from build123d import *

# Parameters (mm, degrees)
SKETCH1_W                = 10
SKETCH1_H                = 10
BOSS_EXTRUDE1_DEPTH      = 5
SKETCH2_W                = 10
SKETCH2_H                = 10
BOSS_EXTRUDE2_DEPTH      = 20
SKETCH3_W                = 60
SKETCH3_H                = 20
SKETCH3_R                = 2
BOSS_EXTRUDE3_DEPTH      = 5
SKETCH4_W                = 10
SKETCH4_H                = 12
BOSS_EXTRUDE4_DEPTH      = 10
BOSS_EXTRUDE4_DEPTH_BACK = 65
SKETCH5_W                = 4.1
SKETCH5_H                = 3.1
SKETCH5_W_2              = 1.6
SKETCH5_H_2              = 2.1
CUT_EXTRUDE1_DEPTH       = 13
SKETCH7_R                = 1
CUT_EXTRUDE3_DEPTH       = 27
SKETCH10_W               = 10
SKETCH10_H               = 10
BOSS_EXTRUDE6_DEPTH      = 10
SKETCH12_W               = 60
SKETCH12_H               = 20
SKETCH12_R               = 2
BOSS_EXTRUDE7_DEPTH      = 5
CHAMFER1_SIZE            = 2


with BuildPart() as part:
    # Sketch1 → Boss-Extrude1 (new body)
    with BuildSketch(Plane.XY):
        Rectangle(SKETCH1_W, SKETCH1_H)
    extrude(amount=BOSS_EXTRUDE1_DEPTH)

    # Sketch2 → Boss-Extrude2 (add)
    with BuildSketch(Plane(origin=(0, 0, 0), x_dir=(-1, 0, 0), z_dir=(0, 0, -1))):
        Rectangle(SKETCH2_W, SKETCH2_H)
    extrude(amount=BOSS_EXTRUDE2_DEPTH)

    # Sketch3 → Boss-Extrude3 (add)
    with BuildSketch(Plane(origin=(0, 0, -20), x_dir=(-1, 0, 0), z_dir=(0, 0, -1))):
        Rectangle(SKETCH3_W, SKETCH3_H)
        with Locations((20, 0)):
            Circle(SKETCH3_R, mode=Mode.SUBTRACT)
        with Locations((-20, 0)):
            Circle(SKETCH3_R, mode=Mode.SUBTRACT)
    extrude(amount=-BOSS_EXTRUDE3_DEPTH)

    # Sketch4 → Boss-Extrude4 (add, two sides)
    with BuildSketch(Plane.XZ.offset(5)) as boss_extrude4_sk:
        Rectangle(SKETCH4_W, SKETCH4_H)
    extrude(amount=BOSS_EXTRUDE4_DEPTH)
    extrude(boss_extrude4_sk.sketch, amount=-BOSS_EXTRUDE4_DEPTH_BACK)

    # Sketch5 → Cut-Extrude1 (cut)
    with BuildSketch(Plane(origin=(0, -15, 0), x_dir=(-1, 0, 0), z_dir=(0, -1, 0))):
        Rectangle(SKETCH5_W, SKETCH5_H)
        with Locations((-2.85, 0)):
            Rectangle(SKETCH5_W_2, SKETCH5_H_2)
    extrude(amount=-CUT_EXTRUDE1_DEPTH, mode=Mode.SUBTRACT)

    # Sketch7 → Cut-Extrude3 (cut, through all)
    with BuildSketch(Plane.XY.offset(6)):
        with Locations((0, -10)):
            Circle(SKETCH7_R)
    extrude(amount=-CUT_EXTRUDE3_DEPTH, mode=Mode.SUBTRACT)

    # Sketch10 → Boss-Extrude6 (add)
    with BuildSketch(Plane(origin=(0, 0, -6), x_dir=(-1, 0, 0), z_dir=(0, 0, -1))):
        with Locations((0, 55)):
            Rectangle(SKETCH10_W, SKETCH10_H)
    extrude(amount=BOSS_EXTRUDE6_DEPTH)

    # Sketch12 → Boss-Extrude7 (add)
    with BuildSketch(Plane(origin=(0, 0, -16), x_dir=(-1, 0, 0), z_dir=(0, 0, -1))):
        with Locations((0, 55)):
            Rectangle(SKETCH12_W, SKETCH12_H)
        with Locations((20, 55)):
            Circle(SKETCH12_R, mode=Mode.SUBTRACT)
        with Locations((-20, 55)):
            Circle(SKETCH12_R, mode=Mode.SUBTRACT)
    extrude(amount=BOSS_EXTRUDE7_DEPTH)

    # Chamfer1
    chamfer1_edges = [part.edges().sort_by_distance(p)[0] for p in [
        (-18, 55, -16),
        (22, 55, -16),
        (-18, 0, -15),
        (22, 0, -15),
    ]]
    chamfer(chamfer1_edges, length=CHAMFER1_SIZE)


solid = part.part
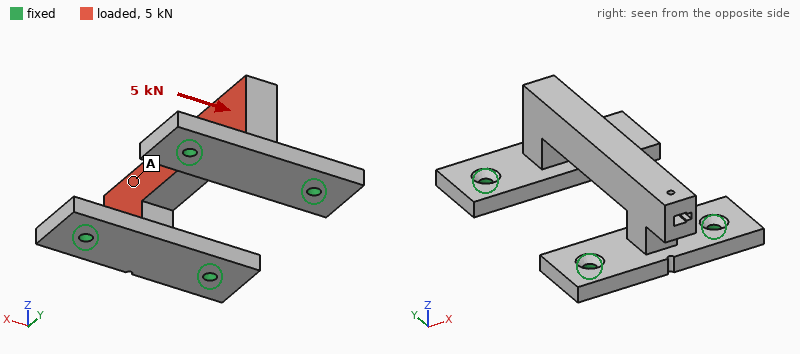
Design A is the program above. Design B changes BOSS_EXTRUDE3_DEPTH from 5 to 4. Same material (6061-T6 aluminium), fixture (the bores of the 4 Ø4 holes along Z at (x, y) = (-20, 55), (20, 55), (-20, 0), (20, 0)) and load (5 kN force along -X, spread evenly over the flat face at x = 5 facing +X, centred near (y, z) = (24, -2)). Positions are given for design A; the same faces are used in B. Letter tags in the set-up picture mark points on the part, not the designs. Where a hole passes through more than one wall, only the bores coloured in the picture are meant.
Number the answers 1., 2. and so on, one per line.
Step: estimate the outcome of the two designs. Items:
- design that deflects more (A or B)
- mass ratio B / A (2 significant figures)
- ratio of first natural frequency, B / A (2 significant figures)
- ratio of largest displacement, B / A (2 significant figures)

1. B
2. 0.95
3. 0.89
4. 1.2
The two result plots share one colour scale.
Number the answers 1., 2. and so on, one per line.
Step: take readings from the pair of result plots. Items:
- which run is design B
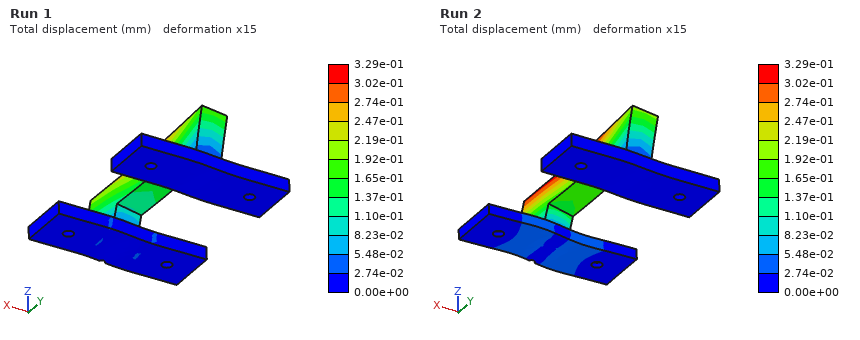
1. Run 2
